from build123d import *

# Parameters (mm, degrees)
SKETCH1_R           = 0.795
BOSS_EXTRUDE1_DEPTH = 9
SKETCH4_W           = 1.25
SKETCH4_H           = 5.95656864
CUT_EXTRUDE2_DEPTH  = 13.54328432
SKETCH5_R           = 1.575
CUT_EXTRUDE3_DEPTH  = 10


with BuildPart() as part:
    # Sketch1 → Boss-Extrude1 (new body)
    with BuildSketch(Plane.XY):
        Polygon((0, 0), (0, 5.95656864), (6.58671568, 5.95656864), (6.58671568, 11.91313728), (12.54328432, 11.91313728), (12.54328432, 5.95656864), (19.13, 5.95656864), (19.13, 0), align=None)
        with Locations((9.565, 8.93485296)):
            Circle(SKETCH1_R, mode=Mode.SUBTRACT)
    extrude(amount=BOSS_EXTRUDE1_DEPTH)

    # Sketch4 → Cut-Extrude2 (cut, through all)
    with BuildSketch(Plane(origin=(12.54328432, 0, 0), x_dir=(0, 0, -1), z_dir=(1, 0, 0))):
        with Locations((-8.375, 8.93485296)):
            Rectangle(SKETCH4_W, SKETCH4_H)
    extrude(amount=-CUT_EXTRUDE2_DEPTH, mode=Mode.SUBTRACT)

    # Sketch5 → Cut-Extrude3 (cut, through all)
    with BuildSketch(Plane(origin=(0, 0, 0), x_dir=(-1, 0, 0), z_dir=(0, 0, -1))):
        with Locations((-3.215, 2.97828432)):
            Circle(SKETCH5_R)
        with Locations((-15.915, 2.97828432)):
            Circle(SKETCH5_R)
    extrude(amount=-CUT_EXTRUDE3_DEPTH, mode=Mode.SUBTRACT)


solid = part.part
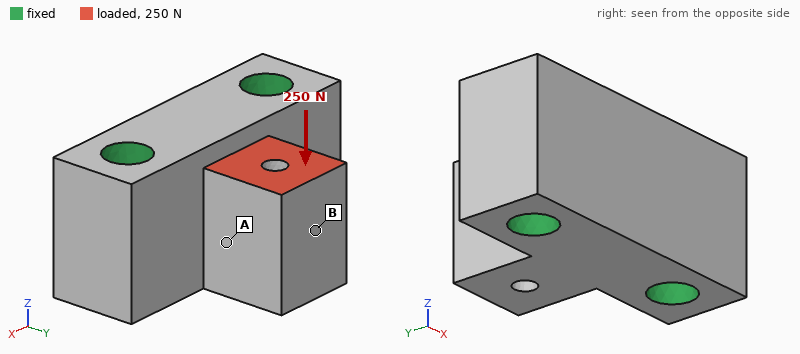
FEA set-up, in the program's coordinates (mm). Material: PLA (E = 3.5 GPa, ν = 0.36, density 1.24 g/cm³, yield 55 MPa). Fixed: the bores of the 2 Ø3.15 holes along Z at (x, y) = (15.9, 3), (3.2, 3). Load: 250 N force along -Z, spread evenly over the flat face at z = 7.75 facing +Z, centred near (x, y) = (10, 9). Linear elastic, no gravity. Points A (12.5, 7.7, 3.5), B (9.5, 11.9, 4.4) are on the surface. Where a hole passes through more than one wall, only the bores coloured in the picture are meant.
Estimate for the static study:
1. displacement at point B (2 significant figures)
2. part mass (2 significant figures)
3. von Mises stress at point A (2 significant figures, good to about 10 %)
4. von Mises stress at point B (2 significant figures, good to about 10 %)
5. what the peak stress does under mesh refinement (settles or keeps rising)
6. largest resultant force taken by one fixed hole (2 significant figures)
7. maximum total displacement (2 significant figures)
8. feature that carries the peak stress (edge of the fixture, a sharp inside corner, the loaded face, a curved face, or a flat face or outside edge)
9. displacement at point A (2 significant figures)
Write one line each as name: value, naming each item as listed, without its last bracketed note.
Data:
displacement at point B: 80 µm
part mass: 1.4 g
von Mises stress at point A: 11 MPa
von Mises stress at point B: 5.0 MPa
what the peak stress does under mesh refinement: keeps rising
largest resultant force taken by one fixed hole: 130 N
maximum total displacement: 92 µm
feature that carries the peak stress: a sharp inside corner
displacement at point A: 40 µm
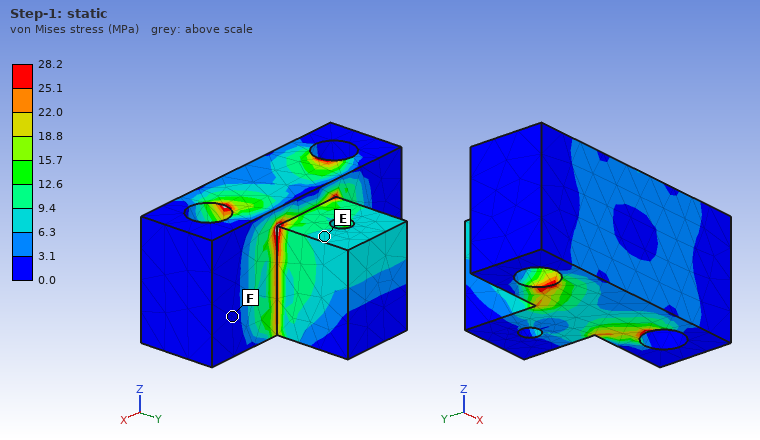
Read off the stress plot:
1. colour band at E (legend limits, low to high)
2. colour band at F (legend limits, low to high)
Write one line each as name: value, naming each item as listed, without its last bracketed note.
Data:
colour band at E: 6.3 to 9.4 MPa
colour band at F: 0.0 to 3.1 MPa
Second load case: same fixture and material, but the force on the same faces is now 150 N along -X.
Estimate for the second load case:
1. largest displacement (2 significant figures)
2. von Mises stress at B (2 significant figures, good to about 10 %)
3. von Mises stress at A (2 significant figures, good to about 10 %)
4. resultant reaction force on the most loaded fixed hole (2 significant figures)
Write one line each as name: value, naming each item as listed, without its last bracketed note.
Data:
largest displacement: 73 µm
von Mises stress at B: 2.7 MPa
von Mises stress at A: 11 MPa
resultant reaction force on the most loaded fixed hole: 110 N
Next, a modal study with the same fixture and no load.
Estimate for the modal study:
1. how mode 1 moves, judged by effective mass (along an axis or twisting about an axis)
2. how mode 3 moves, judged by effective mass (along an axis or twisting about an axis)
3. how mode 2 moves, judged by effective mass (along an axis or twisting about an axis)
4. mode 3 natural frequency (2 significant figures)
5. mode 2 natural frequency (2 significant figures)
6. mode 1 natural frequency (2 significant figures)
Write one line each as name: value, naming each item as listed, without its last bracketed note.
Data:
how mode 1 moves, judged by effective mass: along Z
how mode 3 moves, judged by effective mass: along Y
how mode 2 moves, judged by effective mass: along X
mode 3 natural frequency: 30 kHz
mode 2 natural frequency: 21 kHz
mode 1 natural frequency: 17 kHz
